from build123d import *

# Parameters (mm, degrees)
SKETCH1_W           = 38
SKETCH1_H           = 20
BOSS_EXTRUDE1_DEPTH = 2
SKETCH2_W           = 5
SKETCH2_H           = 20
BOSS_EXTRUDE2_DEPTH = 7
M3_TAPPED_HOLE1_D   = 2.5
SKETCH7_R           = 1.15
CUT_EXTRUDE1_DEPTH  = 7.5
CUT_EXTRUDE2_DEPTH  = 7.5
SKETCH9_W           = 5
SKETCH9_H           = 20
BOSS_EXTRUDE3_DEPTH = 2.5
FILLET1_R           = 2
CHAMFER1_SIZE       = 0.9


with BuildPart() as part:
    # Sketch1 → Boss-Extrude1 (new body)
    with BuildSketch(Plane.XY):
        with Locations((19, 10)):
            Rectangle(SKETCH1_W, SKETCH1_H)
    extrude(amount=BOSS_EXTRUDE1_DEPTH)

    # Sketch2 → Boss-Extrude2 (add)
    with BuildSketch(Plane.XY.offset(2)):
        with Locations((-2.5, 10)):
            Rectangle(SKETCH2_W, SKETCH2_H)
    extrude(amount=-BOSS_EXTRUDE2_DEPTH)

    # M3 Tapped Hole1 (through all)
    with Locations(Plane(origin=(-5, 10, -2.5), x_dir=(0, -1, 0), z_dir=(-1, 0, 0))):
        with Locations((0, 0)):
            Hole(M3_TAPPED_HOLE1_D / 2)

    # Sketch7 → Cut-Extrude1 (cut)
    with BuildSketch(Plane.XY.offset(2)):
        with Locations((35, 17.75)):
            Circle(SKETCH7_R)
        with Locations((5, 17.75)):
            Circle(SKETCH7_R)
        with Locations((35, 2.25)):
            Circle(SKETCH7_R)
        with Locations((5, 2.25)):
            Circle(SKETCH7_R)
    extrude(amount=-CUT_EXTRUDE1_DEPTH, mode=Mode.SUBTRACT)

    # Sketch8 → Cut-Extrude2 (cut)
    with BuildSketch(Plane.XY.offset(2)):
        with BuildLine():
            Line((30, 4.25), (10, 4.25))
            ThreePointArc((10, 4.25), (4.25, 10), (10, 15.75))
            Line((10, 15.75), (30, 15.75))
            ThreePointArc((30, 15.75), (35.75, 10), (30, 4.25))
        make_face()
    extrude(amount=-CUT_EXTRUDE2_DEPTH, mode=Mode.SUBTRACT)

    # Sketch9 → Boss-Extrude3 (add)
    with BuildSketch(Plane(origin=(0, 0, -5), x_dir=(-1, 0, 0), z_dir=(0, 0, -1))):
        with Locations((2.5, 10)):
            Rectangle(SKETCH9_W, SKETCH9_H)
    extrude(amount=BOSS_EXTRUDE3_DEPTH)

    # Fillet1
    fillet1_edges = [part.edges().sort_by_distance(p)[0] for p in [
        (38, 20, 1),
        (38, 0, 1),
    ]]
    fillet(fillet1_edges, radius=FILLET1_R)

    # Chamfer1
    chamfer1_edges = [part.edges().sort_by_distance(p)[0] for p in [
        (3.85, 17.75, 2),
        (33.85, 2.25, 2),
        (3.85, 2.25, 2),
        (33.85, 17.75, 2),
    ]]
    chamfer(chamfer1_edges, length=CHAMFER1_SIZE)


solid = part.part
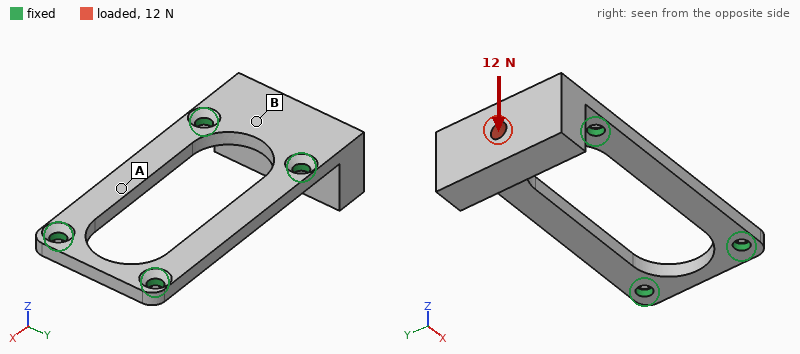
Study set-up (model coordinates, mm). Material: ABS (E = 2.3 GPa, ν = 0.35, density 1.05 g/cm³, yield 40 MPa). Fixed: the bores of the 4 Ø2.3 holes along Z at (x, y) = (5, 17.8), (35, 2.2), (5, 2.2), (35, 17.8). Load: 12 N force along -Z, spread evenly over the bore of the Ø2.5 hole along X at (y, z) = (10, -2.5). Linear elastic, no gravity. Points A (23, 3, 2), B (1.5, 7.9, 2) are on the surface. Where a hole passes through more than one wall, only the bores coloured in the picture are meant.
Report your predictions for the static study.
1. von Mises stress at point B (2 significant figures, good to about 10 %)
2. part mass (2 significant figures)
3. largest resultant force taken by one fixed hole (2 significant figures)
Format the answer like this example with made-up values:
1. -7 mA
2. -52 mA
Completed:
1. 2.5 MPa
2. 1.8 g
3. 6.2 N
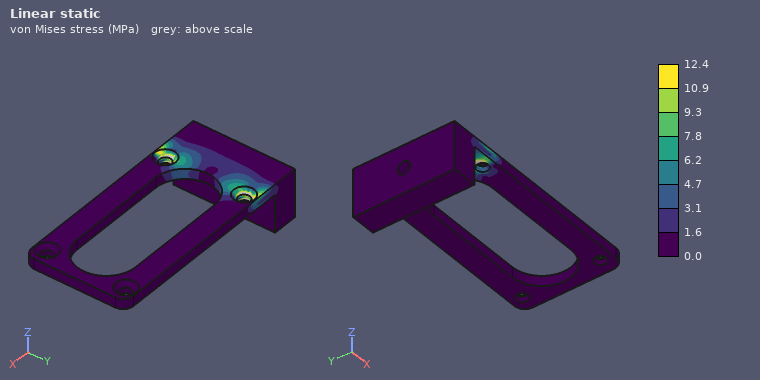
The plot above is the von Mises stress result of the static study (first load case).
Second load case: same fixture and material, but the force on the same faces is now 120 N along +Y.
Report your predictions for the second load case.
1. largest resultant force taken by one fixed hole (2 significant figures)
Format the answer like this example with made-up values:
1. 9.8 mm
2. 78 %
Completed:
1. 82 N
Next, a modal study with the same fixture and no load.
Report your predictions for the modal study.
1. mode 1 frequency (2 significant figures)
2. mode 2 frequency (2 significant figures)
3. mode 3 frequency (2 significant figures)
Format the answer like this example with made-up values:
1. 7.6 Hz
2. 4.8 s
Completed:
1. 1300 Hz
2. 3300 Hz
3. 3300 Hz
